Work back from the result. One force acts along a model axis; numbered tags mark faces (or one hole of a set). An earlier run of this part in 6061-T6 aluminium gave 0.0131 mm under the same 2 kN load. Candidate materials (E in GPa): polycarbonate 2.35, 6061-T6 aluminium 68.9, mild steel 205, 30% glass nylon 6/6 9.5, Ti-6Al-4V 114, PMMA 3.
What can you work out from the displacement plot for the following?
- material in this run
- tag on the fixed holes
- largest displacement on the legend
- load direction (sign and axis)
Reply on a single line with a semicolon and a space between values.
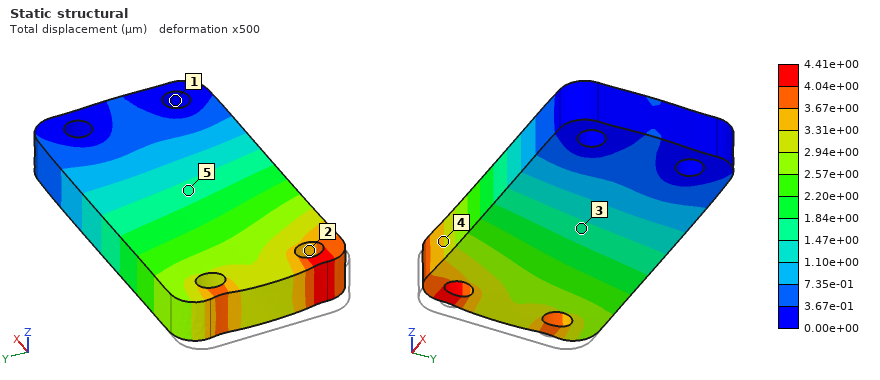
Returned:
mild steel; 1; 4.41e+00 µm; +X
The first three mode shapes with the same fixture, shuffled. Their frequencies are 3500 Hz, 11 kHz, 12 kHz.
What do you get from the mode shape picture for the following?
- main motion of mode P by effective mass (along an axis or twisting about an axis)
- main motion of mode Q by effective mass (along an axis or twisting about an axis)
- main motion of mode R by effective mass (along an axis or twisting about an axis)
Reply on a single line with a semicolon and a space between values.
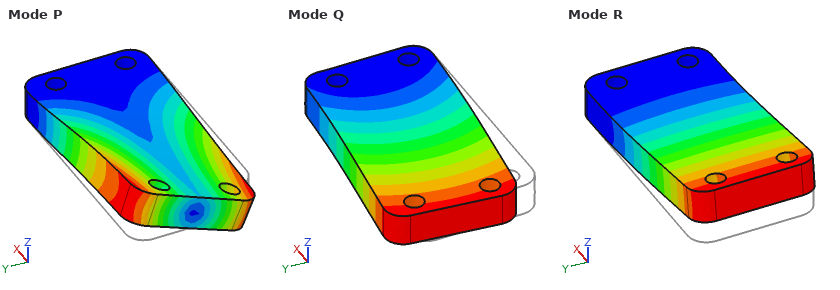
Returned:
twisting about X; along Y; along Z
